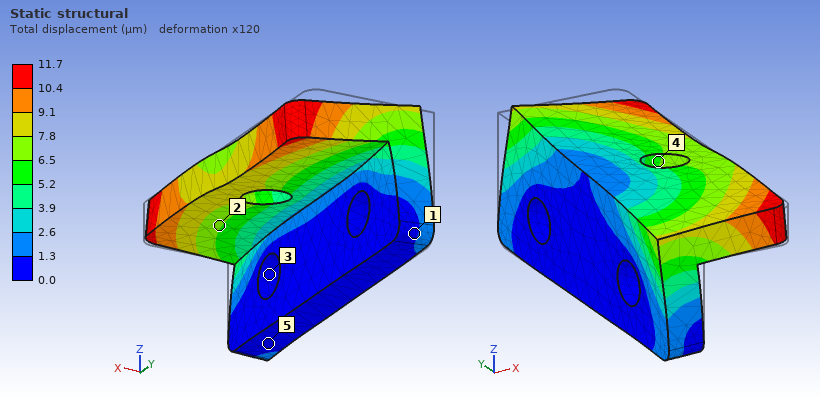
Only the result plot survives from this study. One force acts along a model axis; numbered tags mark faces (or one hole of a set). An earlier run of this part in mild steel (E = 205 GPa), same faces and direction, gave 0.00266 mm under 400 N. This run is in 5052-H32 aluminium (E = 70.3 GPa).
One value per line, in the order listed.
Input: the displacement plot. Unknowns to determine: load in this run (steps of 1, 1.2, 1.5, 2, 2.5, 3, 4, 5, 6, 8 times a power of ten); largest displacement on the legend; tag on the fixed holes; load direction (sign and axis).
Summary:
600 N
11.7 µm
3
-Y
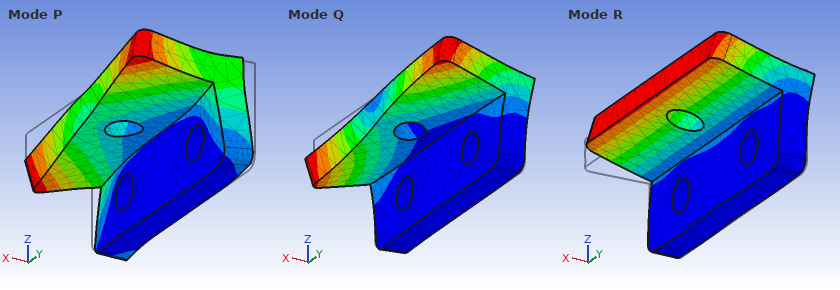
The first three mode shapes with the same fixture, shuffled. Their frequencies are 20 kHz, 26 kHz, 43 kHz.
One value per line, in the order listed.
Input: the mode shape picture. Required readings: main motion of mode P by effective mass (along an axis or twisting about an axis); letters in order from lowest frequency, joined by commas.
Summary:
along Y
R, Q, P
